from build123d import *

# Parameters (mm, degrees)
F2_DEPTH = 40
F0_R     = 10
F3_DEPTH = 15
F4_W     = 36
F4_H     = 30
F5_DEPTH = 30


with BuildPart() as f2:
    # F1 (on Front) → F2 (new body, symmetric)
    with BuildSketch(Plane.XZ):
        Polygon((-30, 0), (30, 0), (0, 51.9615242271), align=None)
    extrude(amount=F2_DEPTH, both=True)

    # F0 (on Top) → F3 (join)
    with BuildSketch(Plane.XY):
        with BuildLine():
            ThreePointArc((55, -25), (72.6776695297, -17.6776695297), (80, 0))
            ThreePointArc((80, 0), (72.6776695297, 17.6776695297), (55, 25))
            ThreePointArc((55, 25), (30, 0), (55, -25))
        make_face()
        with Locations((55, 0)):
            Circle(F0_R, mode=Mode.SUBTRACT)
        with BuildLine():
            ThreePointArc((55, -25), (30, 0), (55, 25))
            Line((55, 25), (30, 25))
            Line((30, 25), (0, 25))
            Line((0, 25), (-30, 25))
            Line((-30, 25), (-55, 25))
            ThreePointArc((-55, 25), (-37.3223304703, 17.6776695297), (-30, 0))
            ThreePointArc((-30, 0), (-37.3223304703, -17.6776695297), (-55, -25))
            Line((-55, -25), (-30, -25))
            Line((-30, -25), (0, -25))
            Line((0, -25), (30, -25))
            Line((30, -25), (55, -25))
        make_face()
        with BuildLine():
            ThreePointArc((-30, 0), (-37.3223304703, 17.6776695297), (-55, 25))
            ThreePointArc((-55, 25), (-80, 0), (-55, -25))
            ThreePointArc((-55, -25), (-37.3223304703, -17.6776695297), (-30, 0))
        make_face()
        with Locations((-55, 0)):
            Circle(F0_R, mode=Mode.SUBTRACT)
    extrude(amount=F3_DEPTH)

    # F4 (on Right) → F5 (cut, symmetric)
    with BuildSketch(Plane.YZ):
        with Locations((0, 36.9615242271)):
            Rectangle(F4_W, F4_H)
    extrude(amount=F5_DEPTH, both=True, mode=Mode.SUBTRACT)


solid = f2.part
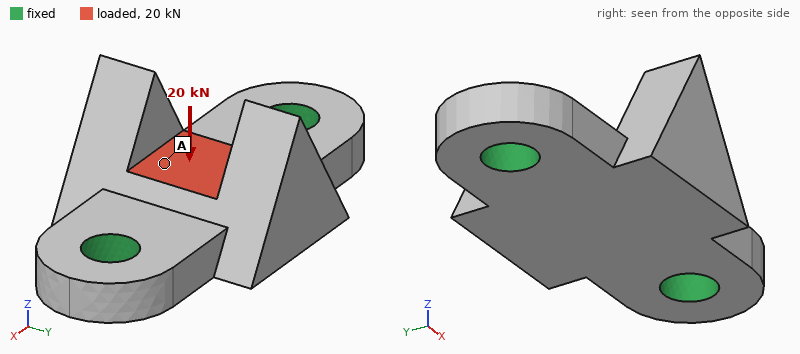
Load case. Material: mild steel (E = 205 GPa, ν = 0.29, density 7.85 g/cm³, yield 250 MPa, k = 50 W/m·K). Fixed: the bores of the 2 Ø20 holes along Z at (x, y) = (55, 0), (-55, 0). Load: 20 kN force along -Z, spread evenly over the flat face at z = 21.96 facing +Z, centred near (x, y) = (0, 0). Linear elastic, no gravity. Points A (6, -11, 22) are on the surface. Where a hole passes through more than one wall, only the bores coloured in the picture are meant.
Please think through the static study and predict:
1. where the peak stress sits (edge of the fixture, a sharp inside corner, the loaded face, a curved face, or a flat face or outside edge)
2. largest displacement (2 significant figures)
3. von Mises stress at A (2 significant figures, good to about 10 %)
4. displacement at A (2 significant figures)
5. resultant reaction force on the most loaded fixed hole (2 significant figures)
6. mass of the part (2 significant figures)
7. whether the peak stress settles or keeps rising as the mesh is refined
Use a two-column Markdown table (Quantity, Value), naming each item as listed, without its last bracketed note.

| Quantity | Value |
|---|---|
| where the peak stress sits | edge of the fixture |
| largest displacement | 22 µm |
| von Mises stress at A | 28 MPa |
| displacement at A | 22 µm |
| resultant reaction force on the most loaded fixed hole | 10 kN |
| mass of the part | 1.3 kg |
| whether the peak stress settles or keeps rising as the mesh is refined | keeps rising |
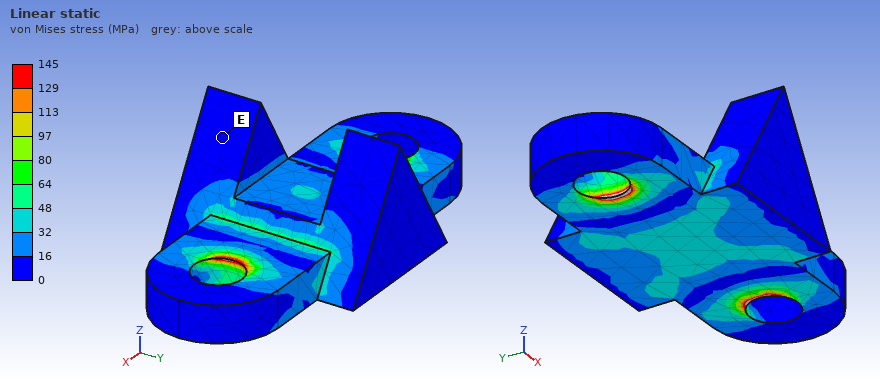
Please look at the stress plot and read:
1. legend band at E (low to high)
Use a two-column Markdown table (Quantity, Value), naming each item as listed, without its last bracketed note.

| Quantity | Value |
|---|---|
| legend band at E | 0 to 16 MPa |
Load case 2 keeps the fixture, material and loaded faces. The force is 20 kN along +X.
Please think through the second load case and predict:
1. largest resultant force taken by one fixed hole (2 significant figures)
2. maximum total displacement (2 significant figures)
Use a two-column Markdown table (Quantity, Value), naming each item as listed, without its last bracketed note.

| Quantity | Value |
|---|---|
| largest resultant force taken by one fixed hole | 11 kN |
| maximum total displacement | 10 µm |
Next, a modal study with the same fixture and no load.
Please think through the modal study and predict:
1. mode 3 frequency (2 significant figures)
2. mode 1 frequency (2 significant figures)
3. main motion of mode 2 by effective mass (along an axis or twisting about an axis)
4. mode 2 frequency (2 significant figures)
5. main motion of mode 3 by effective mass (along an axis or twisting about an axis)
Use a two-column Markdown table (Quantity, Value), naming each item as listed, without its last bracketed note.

| Quantity | Value |
|---|---|
| mode 3 frequency | 8800 Hz |
| mode 1 frequency | 3400 Hz |
| main motion of mode 2 by effective mass | along Z |
| mode 2 frequency | 5000 Hz |
| main motion of mode 3 by effective mass | along Y |
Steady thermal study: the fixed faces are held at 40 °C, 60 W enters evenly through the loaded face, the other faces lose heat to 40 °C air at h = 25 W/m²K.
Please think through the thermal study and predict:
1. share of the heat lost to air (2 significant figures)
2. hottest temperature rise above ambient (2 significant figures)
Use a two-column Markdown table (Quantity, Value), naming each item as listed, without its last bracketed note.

| Quantity | Value |
|---|---|
| share of the heat lost to air | 16 % |
| hottest temperature rise above ambient | 35 K |
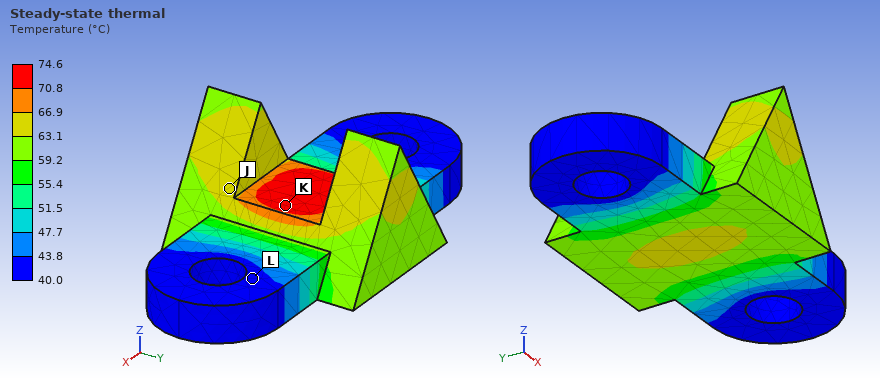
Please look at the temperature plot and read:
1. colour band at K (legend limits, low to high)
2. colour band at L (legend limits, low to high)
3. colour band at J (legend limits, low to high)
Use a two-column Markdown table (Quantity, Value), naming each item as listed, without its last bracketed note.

| Quantity | Value |
|---|---|
| colour band at K | 70.8 to 74.6 °C |
| colour band at L | 40.0 to 43.8 °C |
| colour band at J | 63.1 to 66.9 °C |
